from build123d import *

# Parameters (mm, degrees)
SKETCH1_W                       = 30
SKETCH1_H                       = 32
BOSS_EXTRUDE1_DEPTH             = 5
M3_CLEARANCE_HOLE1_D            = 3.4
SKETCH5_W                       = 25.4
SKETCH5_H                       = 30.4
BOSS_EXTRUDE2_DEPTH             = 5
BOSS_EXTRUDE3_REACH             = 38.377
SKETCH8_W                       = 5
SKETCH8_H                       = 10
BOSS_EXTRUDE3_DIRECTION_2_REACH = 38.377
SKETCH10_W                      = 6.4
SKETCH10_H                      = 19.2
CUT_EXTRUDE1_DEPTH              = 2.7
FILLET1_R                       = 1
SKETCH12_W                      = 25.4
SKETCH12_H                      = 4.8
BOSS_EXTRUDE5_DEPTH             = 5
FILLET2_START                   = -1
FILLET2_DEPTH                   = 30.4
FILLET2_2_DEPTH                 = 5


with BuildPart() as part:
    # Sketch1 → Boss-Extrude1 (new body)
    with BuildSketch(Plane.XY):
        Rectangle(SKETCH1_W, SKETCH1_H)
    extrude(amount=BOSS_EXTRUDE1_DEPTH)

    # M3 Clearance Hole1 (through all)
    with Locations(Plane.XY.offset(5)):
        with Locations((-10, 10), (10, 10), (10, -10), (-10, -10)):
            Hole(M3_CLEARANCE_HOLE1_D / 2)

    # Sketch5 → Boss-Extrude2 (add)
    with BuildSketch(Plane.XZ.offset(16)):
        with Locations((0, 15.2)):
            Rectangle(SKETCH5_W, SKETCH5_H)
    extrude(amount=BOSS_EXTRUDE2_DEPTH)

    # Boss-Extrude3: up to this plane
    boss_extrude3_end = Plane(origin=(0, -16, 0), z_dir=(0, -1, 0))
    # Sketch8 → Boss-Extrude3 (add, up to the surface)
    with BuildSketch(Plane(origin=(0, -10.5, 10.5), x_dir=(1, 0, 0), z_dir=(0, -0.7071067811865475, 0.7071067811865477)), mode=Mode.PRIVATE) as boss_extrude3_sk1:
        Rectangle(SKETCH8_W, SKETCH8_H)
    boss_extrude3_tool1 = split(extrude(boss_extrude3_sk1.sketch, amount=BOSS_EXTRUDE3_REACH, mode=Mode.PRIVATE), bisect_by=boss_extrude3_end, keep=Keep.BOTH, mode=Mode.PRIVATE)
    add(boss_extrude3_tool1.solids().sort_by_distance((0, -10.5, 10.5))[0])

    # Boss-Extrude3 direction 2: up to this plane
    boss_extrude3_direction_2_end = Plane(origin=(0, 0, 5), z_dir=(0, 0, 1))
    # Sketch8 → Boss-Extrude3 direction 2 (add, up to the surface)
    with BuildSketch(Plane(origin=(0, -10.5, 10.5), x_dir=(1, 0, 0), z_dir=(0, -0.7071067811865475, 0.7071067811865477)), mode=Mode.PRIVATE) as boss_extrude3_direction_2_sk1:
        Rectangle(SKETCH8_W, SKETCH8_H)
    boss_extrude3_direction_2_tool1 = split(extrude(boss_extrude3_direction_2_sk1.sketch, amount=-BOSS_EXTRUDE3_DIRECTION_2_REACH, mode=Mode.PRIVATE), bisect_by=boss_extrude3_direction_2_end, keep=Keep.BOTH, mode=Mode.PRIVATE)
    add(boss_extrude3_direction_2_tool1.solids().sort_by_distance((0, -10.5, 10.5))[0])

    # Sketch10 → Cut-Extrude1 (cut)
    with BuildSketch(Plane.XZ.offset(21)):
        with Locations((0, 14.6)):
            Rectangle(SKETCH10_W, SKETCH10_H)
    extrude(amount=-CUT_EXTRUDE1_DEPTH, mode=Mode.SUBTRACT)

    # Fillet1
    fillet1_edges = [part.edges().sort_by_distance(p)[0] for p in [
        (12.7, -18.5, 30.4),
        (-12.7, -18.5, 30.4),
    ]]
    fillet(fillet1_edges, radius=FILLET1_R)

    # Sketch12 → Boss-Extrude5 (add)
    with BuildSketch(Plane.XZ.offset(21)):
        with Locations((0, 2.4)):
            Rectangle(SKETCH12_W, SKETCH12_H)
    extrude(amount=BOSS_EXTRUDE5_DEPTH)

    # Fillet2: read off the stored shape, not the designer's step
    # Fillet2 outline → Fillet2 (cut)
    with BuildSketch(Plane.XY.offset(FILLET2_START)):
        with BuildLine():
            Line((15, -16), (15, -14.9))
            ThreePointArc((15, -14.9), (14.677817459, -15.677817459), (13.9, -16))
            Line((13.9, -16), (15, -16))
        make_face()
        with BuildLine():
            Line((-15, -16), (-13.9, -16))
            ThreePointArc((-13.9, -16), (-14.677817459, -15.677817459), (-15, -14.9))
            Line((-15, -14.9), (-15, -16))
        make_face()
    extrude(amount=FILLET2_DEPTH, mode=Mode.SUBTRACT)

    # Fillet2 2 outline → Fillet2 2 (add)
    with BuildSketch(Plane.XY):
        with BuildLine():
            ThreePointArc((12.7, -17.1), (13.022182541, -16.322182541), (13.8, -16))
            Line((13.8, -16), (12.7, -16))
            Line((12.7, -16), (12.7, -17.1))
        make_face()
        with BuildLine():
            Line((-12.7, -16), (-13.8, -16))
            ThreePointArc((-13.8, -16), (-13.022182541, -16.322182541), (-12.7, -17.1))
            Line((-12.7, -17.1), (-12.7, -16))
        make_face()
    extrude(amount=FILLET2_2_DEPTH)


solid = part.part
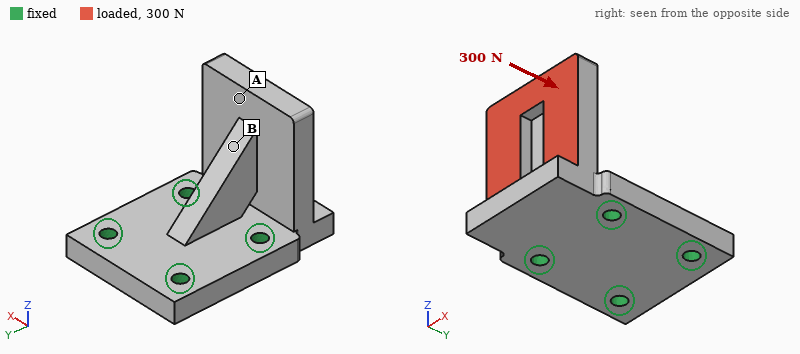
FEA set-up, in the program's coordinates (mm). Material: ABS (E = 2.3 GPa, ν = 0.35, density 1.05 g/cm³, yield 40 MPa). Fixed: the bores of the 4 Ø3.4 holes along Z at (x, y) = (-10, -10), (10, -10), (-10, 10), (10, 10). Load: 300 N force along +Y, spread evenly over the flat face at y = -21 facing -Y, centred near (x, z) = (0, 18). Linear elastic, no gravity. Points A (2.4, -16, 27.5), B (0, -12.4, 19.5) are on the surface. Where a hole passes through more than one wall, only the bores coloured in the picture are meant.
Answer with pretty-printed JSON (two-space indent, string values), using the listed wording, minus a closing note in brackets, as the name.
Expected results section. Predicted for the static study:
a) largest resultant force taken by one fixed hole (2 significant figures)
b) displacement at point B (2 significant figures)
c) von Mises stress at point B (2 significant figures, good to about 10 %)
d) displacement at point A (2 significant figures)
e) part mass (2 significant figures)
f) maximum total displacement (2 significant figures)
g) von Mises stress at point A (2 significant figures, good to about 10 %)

{
  "largest resultant force taken by one fixed hole": "120 N",
  "displacement at point B": "0.28 mm",
  "von Mises stress at point B": "14 MPa",
  "displacement at point A": "0.52 mm",
  "part mass": "10 g",
  "maximum total displacement": "0.68 mm",
  "von Mises stress at point A": "4.2 MPa"
}
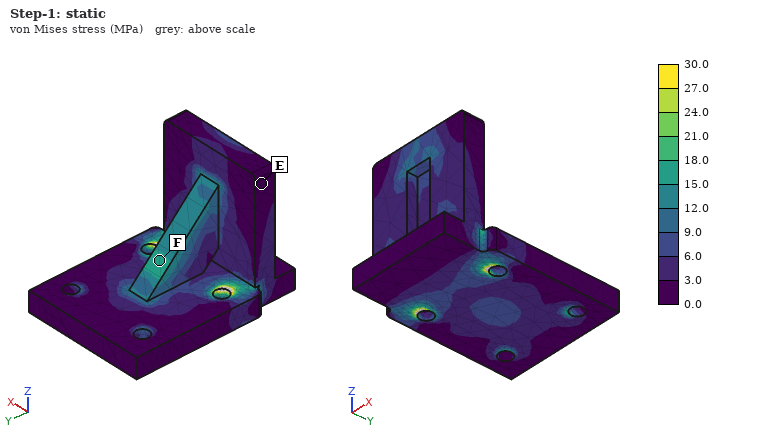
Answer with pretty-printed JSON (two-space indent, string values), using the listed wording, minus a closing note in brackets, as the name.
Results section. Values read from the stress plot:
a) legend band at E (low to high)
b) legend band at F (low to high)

{
  "legend band at E": "0.0 to 3.0 MPa",
  "legend band at F": "15.0 to 18.0 MPa"
}
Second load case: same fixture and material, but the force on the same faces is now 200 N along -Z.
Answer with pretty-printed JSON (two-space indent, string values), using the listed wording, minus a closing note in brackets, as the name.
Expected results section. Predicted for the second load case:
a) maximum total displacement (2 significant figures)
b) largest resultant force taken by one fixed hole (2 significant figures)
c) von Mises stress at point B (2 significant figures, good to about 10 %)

{
  "maximum total displacement": "0.26 mm",
  "largest resultant force taken by one fixed hole": "130 N",
  "von Mises stress at point B": "3.0 MPa"
}
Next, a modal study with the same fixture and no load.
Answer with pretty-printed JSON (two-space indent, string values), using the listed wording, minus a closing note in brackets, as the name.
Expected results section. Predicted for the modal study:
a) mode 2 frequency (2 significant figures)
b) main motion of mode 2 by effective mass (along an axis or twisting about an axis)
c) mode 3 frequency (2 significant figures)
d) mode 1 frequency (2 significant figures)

{
  "mode 2 frequency": "3000 Hz",
  "main motion of mode 2 by effective mass": "along X",
  "mode 3 frequency": "3500 Hz",
  "mode 1 frequency": "2200 Hz"
}
